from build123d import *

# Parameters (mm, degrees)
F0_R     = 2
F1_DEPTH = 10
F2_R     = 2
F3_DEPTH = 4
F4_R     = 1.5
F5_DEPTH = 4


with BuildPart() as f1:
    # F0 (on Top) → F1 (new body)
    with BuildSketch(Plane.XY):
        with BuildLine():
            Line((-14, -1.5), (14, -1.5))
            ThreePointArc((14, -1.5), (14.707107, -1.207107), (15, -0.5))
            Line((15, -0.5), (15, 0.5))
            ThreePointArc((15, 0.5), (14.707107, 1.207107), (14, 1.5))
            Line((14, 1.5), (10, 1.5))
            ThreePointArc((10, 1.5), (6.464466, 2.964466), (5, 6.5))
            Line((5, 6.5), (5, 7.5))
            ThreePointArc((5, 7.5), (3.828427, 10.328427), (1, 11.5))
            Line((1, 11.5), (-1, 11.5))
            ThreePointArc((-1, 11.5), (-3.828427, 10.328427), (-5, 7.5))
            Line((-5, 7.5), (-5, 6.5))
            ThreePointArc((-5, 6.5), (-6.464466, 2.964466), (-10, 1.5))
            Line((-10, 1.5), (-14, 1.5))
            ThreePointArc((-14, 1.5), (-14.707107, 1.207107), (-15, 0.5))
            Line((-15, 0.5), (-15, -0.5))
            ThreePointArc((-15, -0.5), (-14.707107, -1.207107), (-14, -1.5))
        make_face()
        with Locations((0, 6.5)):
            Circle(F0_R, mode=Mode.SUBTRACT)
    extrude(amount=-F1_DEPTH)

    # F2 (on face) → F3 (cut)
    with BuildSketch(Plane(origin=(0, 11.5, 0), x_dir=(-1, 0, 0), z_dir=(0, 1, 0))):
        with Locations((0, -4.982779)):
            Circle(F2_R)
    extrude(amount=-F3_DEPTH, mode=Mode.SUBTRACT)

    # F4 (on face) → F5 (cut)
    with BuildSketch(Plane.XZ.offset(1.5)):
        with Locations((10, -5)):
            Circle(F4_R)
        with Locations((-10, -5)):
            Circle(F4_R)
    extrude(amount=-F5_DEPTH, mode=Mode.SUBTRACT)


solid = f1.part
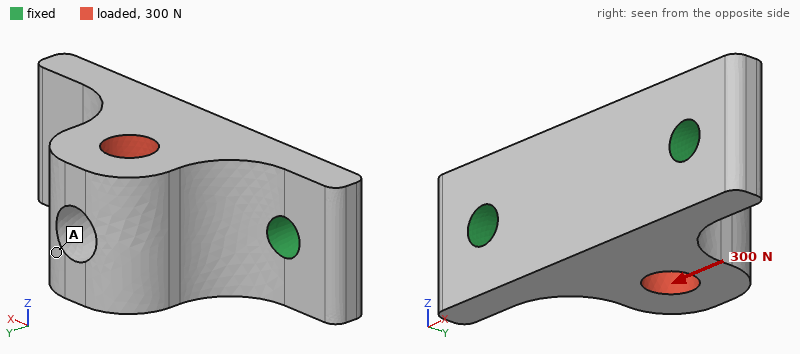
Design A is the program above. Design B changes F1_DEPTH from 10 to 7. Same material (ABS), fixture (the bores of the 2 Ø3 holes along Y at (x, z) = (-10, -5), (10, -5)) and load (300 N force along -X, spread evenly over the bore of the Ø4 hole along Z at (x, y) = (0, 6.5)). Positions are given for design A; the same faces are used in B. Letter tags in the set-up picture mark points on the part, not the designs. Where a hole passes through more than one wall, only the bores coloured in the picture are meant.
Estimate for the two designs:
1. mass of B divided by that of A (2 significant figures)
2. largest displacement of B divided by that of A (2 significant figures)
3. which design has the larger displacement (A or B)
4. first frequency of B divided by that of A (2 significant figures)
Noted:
0.69
1.4
B
0.98
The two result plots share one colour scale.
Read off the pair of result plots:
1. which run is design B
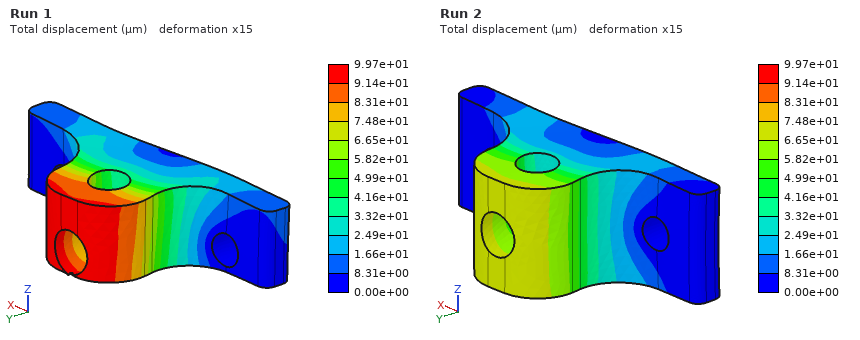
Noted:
Run 1
